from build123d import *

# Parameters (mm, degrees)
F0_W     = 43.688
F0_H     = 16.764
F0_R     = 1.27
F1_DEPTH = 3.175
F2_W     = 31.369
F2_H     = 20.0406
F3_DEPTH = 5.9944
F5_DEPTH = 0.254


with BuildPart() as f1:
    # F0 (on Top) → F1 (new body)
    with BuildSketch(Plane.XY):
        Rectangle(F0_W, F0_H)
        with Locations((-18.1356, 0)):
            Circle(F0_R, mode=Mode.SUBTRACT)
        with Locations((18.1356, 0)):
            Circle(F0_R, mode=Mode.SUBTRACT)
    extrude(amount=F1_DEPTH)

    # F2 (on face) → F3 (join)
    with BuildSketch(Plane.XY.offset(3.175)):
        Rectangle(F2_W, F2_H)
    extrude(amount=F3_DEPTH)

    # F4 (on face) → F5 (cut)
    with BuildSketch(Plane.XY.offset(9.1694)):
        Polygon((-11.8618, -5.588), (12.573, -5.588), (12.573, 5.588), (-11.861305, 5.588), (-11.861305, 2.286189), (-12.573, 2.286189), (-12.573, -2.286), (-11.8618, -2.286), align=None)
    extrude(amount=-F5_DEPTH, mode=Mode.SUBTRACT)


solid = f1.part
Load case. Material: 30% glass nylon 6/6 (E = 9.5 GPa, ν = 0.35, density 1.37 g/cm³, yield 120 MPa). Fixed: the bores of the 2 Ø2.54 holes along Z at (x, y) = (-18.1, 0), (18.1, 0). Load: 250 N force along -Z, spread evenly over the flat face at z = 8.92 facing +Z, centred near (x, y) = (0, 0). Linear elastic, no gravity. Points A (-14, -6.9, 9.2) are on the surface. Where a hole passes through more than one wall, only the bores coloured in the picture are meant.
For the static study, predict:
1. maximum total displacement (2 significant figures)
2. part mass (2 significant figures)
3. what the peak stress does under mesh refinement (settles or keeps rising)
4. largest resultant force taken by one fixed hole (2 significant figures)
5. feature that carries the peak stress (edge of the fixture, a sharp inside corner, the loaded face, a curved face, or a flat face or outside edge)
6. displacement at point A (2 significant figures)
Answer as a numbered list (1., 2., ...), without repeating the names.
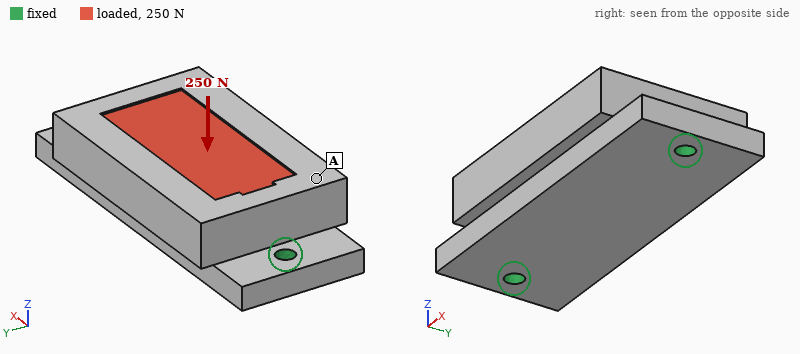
1. 18 µm
2. 8.2 g
3. keeps rising
4. 160 N
5. edge of the fixture
6. 9.9 µm
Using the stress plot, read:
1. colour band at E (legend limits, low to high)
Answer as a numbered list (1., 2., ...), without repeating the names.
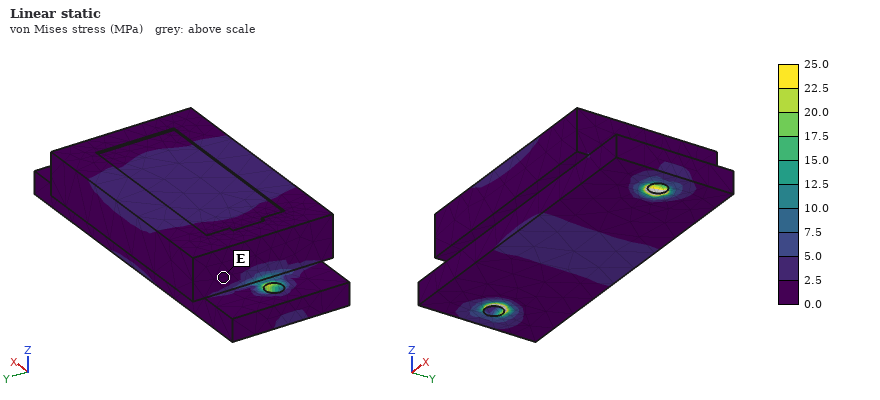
1. 0.0 to 2.5 MPa
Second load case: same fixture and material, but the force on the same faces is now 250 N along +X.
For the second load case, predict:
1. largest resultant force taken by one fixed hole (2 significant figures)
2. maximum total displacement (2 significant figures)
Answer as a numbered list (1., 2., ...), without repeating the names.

1. 140 N
2. 5.2 µm
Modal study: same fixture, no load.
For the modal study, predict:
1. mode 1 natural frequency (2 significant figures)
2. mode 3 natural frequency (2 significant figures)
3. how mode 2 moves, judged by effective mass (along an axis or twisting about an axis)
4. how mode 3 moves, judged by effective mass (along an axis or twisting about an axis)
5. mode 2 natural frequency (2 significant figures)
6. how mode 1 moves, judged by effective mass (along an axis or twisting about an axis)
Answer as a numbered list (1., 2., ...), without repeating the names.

1. 4300 Hz
2. 12 kHz
3. along Z
4. along Y
5. 8000 Hz
6. along Y
